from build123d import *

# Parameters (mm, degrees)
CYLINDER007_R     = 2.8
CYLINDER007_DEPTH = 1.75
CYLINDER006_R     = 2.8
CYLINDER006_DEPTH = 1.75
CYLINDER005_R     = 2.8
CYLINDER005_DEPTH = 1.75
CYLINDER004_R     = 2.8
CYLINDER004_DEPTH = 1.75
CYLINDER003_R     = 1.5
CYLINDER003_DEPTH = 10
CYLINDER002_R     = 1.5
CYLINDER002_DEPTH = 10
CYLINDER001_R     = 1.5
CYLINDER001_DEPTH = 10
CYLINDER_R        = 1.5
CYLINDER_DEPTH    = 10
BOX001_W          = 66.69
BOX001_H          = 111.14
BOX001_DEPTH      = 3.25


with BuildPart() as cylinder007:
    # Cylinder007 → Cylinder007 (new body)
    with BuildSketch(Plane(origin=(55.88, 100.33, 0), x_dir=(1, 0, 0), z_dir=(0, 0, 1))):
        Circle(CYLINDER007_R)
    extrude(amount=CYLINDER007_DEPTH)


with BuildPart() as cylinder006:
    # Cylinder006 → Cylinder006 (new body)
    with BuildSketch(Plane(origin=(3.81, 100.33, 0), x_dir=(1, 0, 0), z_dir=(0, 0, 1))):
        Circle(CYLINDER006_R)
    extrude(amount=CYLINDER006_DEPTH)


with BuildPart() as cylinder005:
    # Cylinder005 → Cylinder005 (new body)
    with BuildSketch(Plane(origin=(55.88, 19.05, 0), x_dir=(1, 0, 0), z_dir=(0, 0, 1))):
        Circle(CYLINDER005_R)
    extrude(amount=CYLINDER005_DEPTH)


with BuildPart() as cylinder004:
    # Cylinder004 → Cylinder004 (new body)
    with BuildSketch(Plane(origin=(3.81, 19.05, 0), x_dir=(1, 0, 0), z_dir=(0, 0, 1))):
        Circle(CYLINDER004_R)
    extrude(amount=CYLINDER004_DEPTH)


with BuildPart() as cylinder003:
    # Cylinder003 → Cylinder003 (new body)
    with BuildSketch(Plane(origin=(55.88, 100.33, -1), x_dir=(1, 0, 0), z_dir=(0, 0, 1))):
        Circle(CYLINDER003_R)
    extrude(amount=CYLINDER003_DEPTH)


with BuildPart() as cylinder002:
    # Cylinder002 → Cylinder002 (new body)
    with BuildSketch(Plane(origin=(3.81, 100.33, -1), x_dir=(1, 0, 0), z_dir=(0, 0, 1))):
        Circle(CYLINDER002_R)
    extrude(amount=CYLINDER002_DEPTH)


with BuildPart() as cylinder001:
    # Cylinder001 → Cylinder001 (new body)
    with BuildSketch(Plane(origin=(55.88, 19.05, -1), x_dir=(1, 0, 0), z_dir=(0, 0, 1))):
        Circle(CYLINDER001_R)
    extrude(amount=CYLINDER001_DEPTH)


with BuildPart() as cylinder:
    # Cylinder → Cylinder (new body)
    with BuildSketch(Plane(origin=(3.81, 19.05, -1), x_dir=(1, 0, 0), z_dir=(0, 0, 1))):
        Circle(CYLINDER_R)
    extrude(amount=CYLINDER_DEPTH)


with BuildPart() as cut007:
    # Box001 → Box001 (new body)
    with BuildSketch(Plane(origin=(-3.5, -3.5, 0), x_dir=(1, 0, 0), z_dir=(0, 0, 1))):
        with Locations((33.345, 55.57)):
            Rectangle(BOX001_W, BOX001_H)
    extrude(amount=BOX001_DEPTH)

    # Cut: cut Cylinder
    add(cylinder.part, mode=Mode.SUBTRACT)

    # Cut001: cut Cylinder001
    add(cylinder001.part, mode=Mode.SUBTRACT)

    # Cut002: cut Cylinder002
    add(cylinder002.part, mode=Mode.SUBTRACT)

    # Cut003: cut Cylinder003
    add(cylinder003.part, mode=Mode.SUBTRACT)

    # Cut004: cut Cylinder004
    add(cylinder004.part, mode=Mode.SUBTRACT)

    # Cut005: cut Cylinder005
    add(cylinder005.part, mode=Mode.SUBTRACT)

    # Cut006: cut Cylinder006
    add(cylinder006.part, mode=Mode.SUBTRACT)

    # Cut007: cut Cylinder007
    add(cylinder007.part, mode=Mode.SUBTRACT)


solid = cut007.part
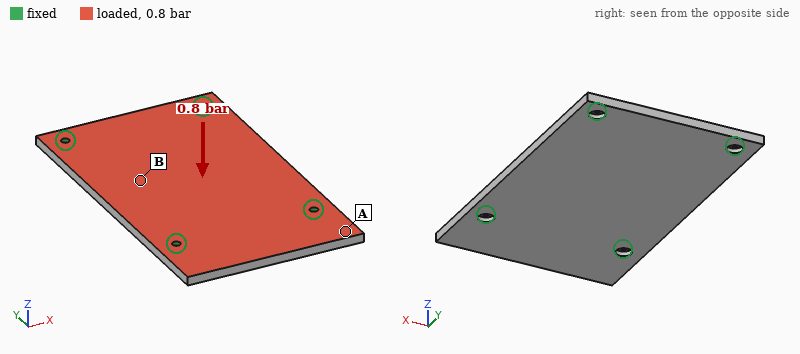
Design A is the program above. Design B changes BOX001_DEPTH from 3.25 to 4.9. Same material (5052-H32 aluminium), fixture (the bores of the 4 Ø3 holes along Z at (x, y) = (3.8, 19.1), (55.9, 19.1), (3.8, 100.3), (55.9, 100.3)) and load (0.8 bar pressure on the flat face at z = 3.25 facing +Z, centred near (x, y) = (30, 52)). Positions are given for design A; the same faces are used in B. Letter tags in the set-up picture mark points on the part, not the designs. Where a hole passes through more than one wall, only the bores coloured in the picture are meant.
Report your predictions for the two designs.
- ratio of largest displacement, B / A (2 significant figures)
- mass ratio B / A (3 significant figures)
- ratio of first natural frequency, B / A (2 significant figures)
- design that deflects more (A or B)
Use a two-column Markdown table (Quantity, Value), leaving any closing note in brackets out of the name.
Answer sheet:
| Quantity | Value |
|---|---|
| ratio of largest displacement, B / A | 0.29 |
| mass ratio B / A | 1.51 |
| ratio of first natural frequency, B / A | 1.5 |
| design that deflects more | A |
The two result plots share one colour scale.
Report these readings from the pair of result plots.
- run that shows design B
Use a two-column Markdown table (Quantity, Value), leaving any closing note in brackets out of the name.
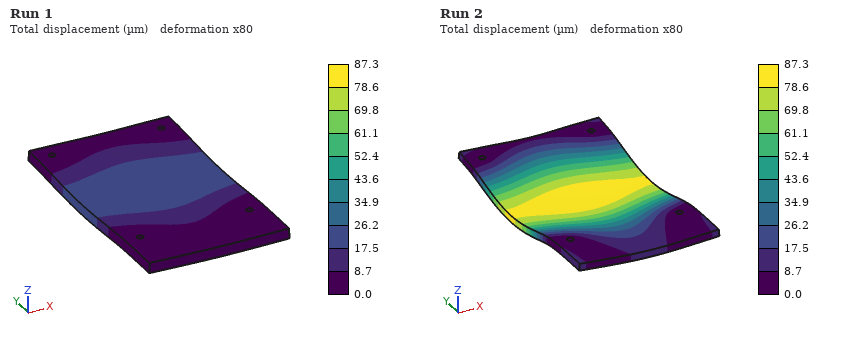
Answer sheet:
| Quantity | Value |
|---|---|
| run that shows design B | Run 1 |
